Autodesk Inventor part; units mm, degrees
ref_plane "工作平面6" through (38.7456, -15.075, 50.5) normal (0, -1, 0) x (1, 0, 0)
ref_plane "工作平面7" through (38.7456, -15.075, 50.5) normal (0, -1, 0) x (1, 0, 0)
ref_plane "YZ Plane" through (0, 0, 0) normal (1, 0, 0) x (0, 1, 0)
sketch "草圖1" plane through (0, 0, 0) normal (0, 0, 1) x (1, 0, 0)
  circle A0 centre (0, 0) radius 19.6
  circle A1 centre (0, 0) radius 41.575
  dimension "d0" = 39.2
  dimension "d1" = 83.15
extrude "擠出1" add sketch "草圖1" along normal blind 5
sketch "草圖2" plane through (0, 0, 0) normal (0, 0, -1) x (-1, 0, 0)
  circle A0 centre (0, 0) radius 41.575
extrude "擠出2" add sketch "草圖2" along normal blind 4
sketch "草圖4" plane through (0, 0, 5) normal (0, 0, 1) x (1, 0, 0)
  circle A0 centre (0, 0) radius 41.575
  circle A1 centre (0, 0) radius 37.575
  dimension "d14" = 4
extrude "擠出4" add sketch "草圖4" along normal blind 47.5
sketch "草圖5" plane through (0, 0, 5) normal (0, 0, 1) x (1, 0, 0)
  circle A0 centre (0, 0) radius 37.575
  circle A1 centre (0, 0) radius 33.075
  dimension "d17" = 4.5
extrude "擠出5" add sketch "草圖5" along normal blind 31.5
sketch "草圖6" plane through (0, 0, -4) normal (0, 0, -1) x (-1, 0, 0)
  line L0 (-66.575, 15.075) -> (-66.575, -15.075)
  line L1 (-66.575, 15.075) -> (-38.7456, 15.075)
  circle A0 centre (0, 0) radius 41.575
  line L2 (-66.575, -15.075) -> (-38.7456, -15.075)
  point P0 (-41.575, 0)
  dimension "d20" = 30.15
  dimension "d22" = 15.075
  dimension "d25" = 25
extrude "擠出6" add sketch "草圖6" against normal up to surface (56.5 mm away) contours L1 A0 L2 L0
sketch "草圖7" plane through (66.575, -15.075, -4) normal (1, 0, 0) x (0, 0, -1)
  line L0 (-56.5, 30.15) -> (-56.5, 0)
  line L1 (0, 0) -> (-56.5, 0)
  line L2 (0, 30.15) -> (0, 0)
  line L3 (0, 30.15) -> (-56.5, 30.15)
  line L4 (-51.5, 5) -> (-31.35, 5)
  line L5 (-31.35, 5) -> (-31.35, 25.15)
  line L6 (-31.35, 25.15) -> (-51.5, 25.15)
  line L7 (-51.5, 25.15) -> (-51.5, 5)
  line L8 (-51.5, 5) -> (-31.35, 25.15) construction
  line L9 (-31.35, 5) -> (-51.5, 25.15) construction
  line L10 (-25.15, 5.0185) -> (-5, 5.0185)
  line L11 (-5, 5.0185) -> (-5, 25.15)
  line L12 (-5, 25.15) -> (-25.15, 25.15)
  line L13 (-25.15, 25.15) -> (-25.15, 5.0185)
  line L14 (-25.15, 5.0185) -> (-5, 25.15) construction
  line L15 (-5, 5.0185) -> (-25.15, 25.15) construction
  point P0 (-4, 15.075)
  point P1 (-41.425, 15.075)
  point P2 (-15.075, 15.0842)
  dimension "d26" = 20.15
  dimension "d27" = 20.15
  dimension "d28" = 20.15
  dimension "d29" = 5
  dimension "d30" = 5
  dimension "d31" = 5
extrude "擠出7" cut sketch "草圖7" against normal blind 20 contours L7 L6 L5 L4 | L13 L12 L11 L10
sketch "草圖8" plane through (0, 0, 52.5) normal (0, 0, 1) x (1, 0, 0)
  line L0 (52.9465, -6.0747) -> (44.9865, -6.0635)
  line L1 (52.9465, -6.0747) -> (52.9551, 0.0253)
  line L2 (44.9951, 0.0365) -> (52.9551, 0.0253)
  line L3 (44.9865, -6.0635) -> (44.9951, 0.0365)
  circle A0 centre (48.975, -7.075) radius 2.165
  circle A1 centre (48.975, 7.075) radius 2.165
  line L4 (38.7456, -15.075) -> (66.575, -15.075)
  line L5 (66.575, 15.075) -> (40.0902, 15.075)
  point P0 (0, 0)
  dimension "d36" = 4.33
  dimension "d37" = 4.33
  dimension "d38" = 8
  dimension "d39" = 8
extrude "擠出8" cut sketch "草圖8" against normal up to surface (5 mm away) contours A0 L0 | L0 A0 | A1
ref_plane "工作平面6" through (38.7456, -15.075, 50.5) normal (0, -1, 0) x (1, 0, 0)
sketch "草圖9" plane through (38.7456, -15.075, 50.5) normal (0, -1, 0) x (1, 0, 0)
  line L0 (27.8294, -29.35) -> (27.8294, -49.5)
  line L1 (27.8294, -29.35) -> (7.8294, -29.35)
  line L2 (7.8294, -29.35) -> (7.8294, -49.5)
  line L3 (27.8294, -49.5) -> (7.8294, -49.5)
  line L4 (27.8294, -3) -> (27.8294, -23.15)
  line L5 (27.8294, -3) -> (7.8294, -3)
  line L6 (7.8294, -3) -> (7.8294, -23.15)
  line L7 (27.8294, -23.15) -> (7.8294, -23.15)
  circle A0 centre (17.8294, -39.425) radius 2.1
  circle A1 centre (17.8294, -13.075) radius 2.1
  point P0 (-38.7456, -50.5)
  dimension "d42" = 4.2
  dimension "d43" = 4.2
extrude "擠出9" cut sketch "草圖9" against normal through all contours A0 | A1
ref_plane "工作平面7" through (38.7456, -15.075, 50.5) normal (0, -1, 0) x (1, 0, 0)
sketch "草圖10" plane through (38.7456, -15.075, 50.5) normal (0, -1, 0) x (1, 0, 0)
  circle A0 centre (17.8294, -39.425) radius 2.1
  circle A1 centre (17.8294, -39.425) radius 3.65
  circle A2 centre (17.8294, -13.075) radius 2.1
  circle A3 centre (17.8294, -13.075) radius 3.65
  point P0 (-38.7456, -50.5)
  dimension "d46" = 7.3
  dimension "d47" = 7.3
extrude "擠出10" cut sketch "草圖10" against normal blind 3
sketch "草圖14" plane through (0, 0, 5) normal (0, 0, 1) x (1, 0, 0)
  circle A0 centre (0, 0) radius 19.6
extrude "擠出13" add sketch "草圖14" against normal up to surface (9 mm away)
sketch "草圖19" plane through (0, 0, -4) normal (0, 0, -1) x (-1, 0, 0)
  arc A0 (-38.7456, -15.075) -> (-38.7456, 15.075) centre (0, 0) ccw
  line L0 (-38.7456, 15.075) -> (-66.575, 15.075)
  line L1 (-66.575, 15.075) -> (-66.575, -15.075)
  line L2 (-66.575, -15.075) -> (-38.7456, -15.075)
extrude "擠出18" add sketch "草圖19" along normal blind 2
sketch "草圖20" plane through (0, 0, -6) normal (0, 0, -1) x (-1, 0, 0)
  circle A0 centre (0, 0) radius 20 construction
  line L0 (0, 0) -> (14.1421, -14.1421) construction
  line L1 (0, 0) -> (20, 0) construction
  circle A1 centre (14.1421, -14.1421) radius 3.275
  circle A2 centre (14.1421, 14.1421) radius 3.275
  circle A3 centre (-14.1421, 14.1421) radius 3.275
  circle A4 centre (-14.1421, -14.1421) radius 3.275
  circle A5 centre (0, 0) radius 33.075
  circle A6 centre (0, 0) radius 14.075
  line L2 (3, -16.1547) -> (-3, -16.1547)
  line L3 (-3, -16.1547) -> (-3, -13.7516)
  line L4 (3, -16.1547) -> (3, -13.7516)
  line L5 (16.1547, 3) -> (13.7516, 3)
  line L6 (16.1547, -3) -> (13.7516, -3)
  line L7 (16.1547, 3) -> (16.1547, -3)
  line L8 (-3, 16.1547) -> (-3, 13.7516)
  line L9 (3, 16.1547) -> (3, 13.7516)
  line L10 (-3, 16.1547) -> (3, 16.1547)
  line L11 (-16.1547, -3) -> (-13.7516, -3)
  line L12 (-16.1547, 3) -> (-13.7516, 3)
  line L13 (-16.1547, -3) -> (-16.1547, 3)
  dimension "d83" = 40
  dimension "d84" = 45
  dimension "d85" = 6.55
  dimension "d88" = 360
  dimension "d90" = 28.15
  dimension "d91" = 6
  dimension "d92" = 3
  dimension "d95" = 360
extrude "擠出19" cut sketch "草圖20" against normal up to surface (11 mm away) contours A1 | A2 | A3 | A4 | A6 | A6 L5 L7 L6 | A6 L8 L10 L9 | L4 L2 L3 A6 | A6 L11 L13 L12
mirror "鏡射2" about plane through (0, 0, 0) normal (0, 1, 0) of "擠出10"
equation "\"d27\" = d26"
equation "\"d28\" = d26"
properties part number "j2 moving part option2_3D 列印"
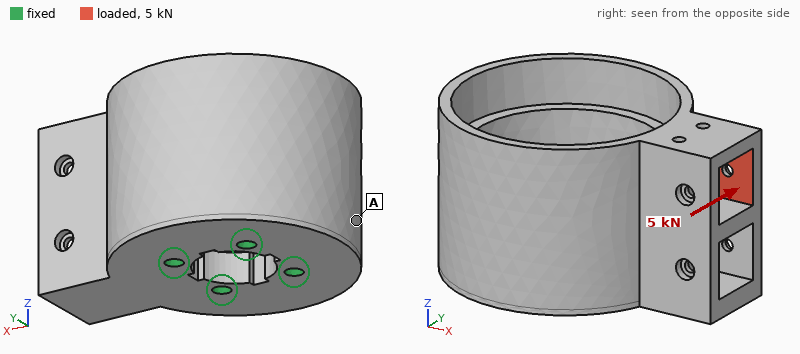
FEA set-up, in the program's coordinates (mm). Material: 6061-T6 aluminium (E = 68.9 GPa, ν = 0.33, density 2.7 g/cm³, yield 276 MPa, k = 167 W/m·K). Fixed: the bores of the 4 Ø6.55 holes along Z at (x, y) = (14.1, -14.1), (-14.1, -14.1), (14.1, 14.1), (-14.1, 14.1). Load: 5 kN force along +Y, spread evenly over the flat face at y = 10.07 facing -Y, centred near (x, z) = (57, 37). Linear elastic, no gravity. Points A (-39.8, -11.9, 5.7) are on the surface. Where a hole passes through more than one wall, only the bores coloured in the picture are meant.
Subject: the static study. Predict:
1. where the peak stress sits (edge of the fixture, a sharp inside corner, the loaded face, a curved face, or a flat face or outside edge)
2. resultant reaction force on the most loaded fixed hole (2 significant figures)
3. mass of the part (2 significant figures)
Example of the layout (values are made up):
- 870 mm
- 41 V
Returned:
- a curved face
- 5.4 kN
- 430 g
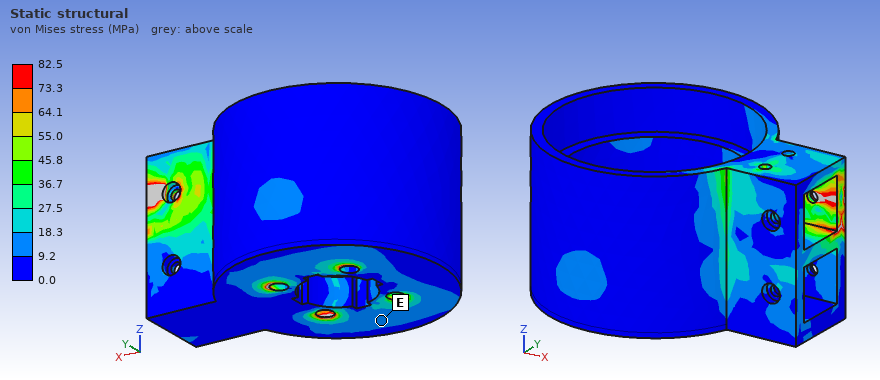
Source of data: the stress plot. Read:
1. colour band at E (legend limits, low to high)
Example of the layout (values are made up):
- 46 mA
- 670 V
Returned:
- 9.2 to 18.3 MPa
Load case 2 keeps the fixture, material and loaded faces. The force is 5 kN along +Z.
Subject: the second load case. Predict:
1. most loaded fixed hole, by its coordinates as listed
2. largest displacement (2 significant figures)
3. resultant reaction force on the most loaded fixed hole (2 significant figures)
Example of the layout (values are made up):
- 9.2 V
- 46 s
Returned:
- (14.1, 14.1)
- 0.19 mm
- 5.2 kN
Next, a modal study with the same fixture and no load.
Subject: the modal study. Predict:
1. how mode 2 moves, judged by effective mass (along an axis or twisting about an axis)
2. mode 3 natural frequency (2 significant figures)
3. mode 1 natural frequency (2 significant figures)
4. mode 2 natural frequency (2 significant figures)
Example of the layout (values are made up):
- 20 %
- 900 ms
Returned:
- along Y
- 4700 Hz
- 3000 Hz
- 4100 Hz
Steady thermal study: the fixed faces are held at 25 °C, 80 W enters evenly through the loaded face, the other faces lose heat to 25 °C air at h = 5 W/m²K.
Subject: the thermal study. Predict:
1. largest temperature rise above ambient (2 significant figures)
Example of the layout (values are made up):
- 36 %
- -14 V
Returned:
- 54 K
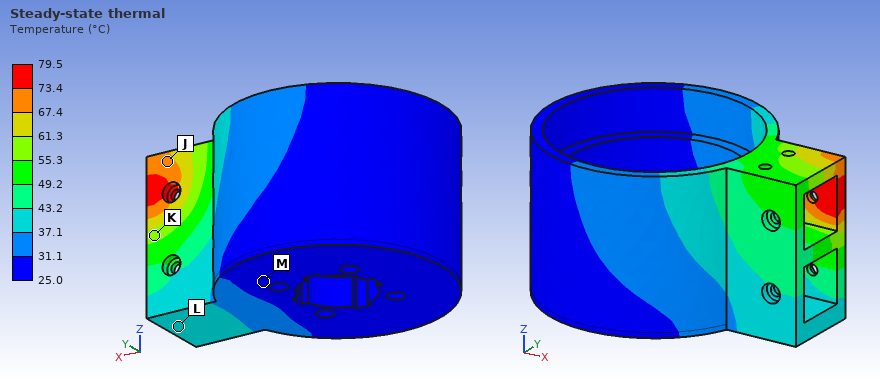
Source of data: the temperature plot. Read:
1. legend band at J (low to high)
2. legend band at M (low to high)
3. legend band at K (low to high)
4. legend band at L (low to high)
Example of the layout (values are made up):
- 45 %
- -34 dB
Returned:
- 67.4 to 73.4 °C
- 25.0 to 31.1 °C
- 55.3 to 61.3 °C
- 37.1 to 43.2 °C
